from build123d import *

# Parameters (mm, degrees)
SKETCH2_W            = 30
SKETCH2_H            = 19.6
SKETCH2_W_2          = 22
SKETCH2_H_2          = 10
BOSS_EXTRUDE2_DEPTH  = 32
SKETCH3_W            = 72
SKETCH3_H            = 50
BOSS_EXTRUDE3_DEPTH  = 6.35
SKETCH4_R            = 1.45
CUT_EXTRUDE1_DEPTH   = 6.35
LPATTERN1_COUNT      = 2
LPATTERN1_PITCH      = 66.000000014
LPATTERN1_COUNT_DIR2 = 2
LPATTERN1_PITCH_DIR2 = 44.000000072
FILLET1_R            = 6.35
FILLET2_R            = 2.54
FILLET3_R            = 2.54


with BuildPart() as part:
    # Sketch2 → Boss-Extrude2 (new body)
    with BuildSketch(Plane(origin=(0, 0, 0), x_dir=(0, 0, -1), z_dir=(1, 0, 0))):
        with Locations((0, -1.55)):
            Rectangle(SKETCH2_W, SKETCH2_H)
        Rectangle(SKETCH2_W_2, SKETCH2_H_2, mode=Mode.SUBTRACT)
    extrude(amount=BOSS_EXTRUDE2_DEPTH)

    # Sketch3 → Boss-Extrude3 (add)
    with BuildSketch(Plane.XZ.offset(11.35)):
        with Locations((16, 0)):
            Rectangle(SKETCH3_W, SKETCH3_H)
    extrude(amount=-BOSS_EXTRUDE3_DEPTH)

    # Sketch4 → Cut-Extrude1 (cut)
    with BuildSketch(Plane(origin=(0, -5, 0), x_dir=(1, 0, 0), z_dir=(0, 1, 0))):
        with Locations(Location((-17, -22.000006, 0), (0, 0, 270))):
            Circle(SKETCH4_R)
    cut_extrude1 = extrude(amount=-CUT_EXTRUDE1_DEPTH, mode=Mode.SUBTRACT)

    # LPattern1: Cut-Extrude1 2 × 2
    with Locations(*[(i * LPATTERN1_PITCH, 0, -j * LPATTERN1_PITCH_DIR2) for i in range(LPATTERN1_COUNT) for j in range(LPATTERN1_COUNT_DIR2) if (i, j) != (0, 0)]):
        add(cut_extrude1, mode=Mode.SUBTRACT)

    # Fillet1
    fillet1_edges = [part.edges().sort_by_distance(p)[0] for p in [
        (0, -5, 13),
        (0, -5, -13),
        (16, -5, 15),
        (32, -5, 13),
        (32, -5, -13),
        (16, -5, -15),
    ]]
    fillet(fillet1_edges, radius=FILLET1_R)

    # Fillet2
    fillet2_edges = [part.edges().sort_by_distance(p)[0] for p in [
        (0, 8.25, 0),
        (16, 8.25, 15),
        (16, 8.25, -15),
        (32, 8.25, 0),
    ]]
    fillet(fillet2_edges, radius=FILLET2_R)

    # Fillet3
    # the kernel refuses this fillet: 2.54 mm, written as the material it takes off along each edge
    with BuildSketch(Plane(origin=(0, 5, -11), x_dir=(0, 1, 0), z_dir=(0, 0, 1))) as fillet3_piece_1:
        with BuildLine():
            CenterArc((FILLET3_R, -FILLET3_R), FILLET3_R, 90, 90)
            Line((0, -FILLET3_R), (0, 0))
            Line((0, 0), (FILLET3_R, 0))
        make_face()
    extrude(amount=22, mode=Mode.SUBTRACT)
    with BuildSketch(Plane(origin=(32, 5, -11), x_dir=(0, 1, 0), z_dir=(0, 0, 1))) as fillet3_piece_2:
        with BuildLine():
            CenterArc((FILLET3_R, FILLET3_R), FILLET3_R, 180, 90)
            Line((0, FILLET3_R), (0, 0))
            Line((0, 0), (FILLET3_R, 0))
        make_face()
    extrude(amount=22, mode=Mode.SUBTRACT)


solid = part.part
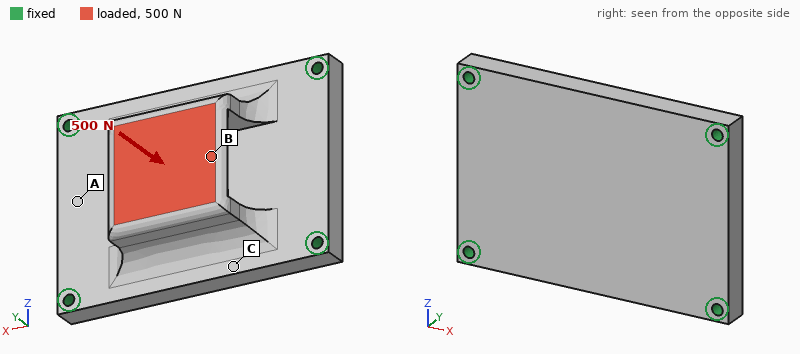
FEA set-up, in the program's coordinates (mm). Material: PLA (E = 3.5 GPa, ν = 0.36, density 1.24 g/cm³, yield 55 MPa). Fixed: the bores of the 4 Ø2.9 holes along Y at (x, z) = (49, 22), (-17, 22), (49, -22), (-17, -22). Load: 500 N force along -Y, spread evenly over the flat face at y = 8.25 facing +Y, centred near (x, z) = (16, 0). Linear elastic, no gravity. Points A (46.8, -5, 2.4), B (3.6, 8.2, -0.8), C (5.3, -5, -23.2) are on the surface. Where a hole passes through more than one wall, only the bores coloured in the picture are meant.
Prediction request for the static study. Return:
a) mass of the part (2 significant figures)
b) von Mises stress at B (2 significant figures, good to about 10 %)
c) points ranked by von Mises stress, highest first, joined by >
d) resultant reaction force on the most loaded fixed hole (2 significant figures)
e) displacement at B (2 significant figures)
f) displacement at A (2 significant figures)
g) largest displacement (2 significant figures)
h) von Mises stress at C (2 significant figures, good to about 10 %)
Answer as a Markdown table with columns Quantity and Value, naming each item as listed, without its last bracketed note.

| Quantity | Value |
|---|---|
| mass of the part | 36 g |
| von Mises stress at B | 11 MPa |
| points ranked by von Mises stress, highest first, joined by > | B > C > A |
| resultant reaction force on the most loaded fixed hole | 140 N |
| displacement at B | 0.21 mm |
| displacement at A | 0.039 mm |
| largest displacement | 0.22 mm |
| von Mises stress at C | 3.5 MPa |
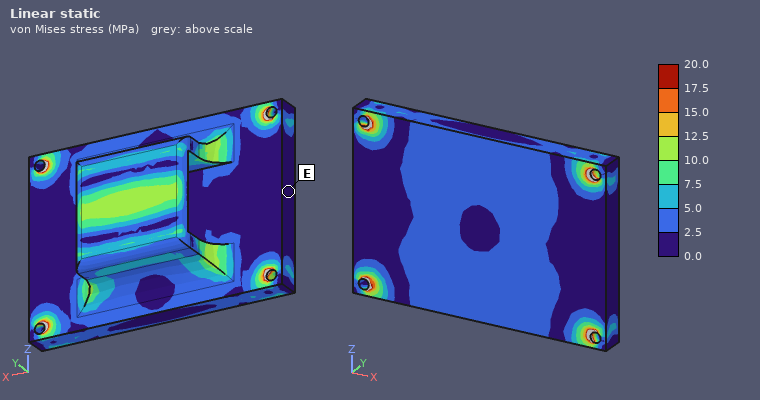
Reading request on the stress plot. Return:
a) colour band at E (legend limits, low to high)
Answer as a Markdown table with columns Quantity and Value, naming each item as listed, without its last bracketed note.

| Quantity | Value |
|---|---|
| colour band at E | 0.0 to 2.5 MPa |
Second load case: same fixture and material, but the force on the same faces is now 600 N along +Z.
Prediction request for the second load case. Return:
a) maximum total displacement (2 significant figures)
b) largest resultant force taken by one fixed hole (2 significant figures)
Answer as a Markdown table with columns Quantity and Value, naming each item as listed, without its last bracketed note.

| Quantity | Value |
|---|---|
| maximum total displacement | 0.25 mm |
| largest resultant force taken by one fixed hole | 230 N |
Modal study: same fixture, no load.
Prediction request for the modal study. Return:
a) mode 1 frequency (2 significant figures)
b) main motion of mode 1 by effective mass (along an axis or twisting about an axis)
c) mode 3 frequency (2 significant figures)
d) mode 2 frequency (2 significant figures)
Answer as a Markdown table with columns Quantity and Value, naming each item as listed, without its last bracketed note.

| Quantity | Value |
|---|---|
| mode 1 frequency | 2000 Hz |
| main motion of mode 1 by effective mass | along Y |
| mode 3 frequency | 4000 Hz |
| mode 2 frequency | 2700 Hz |
